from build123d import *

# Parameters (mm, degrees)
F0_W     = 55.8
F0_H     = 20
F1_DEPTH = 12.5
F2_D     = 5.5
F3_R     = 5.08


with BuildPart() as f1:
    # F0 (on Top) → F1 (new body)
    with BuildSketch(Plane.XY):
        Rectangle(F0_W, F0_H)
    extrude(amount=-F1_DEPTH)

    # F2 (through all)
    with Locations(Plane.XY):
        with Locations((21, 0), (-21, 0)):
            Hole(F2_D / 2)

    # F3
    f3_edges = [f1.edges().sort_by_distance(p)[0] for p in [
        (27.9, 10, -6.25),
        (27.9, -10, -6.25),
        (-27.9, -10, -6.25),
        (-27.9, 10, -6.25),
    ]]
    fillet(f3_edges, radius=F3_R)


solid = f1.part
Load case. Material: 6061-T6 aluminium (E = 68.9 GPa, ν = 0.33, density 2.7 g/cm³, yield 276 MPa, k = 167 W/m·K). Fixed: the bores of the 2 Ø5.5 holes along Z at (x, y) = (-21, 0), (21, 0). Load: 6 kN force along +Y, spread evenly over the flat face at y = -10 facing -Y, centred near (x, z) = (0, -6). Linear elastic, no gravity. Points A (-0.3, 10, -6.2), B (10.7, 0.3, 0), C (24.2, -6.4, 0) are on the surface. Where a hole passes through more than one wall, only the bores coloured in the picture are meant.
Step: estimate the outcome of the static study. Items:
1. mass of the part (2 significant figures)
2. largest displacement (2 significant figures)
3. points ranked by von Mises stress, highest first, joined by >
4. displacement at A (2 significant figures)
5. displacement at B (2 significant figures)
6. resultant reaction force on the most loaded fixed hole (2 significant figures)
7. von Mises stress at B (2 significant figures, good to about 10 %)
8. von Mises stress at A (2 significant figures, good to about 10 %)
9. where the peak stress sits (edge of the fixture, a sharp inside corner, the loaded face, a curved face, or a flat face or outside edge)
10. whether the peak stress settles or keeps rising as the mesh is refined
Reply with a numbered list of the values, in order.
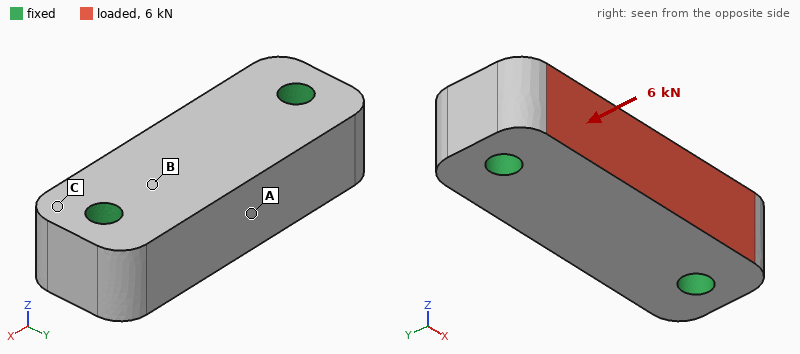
1. 35 g
2. 9.6 µm
3. A > B > C
4. 7.9 µm
5. 5.9 µm
6. 3.0 kN
7. 15 MPa
8. 22 MPa
9. edge of the fixture
10. keeps rising
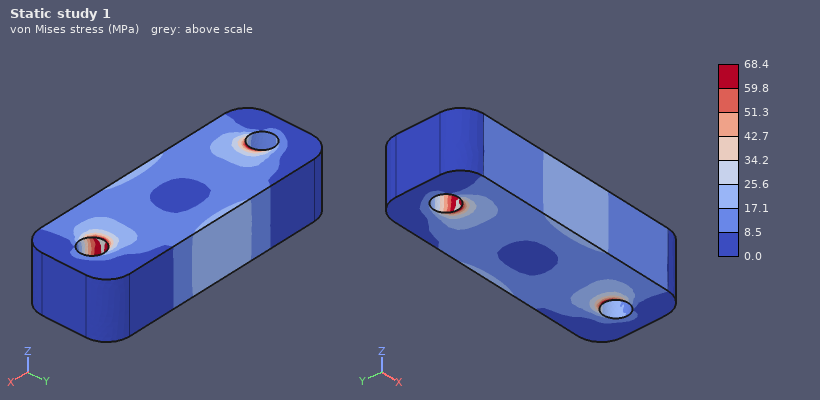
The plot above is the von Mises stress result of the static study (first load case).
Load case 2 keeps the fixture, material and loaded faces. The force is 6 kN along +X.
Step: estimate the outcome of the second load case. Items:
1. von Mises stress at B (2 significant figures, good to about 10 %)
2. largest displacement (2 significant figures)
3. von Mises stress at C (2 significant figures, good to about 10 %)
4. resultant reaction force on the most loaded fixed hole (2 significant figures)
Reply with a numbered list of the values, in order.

1. 11 MPa
2. 5.0 µm
3. 11 MPa
4. 3.2 kN
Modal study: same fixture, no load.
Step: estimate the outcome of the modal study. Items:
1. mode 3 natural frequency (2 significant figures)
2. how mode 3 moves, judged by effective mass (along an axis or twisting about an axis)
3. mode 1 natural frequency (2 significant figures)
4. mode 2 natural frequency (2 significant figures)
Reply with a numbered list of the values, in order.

1. 30 kHz
2. twisting about X
3. 25 kHz
4. 26 kHz
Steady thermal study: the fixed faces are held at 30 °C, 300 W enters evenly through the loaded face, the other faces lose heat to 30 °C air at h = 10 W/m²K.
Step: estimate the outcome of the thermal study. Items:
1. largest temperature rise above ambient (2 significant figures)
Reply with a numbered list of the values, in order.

1. 57 K
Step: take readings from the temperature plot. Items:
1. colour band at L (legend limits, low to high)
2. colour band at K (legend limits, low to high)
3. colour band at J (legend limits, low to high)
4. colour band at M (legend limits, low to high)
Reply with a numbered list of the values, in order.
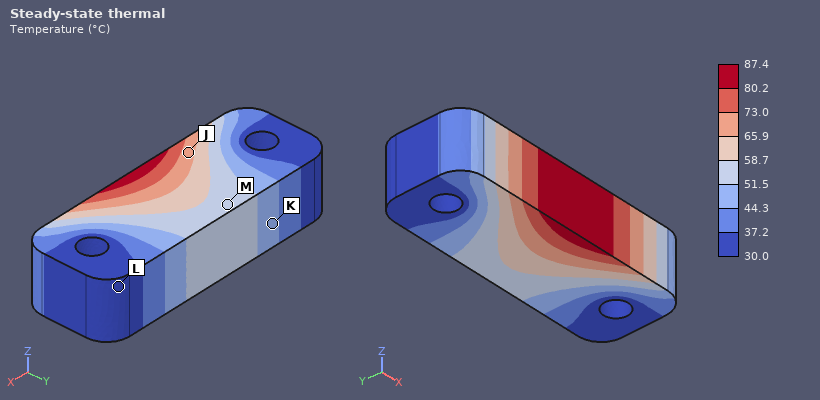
1. 30.0 to 37.2 °C
2. 44.3 to 51.5 °C
3. 65.9 to 73.0 °C
4. 51.5 to 58.7 °C
